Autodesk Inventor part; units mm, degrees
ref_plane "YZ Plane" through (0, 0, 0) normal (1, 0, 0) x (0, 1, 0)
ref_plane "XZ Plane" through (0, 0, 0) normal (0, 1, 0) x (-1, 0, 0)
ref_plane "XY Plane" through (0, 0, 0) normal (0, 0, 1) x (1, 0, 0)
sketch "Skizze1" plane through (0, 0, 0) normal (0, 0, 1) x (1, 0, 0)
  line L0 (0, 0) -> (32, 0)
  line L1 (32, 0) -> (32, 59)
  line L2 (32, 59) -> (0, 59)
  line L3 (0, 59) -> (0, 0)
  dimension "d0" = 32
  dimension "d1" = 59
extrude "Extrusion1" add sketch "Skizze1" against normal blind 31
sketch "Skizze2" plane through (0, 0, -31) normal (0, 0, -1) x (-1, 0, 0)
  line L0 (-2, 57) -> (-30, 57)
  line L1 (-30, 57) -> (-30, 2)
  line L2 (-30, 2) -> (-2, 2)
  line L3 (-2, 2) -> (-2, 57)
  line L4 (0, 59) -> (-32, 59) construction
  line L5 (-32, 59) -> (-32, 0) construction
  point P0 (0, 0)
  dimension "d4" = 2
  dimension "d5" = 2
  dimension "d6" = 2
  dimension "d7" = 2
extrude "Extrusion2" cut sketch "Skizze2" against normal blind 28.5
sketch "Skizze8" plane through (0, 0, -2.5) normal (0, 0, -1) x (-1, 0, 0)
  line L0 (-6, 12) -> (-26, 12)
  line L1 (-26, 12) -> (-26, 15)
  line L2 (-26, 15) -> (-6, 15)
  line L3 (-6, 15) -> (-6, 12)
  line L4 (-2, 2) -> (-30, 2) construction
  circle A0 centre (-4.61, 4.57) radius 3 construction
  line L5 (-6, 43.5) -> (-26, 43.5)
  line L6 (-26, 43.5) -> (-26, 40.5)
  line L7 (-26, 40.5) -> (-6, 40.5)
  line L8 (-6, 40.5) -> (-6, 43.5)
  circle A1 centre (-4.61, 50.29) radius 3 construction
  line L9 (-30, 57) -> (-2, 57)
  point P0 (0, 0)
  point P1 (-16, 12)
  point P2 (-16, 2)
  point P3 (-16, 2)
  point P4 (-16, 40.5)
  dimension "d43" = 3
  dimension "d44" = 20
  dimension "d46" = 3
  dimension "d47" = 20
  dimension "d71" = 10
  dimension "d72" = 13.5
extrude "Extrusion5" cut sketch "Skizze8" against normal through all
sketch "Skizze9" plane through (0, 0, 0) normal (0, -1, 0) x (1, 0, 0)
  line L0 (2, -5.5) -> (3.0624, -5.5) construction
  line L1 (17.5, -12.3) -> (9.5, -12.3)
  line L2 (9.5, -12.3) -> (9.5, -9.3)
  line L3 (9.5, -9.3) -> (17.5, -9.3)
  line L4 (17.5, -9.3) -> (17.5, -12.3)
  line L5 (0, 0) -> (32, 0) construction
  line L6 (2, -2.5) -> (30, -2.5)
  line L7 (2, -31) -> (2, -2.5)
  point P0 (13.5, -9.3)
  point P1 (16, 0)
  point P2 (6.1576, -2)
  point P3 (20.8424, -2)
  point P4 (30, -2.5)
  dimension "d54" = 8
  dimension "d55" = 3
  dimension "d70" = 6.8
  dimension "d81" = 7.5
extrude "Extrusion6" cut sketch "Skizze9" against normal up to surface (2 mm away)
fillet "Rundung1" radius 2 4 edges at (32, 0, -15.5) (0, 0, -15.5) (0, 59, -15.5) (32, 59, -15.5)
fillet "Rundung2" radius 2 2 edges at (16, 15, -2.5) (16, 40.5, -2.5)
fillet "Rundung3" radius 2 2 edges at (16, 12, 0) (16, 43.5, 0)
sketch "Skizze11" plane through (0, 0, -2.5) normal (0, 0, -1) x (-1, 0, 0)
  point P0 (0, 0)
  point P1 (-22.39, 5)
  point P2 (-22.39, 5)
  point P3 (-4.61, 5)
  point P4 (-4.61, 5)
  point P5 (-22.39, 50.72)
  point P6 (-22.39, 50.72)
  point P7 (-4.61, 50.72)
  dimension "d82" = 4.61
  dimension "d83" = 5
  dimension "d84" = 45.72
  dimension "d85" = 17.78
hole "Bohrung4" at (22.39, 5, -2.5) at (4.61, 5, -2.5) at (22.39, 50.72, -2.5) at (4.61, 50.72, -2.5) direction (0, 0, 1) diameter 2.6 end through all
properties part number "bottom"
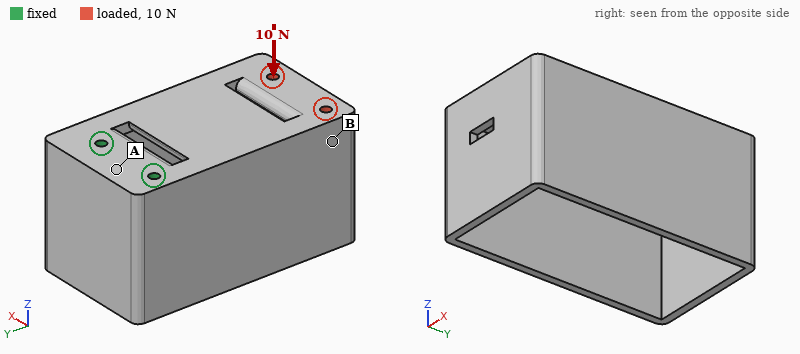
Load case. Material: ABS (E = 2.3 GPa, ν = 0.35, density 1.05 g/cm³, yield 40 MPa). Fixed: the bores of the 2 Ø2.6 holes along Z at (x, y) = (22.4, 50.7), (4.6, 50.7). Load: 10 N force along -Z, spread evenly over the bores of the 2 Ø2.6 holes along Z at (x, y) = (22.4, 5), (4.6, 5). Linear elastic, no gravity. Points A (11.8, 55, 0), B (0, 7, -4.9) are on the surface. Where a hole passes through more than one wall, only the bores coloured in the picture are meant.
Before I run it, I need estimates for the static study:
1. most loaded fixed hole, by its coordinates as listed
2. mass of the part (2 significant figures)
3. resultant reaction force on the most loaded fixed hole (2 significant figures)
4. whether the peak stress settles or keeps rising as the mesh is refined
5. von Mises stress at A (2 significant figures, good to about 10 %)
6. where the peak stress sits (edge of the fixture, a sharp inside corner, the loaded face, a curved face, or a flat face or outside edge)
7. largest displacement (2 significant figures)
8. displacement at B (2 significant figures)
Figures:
(4.6, 50.7)
15 g
6.5 N
keeps rising
2.2 MPa
edge of the fixture
0.78 mm
0.54 mm
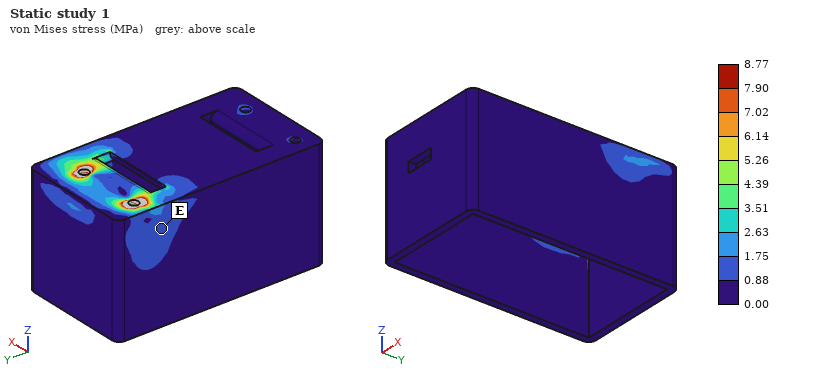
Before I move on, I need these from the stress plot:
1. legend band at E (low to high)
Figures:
0.88 to 1.75 MPa
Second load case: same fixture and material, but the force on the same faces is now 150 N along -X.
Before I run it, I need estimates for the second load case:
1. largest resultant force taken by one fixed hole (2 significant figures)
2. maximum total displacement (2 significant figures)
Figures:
360 N
0.88 mm
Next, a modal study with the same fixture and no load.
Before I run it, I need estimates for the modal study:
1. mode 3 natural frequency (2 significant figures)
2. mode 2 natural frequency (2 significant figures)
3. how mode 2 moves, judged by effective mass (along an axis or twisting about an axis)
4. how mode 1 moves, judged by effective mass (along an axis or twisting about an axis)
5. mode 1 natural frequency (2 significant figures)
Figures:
960 Hz
410 Hz
along X
along Z
240 Hz
